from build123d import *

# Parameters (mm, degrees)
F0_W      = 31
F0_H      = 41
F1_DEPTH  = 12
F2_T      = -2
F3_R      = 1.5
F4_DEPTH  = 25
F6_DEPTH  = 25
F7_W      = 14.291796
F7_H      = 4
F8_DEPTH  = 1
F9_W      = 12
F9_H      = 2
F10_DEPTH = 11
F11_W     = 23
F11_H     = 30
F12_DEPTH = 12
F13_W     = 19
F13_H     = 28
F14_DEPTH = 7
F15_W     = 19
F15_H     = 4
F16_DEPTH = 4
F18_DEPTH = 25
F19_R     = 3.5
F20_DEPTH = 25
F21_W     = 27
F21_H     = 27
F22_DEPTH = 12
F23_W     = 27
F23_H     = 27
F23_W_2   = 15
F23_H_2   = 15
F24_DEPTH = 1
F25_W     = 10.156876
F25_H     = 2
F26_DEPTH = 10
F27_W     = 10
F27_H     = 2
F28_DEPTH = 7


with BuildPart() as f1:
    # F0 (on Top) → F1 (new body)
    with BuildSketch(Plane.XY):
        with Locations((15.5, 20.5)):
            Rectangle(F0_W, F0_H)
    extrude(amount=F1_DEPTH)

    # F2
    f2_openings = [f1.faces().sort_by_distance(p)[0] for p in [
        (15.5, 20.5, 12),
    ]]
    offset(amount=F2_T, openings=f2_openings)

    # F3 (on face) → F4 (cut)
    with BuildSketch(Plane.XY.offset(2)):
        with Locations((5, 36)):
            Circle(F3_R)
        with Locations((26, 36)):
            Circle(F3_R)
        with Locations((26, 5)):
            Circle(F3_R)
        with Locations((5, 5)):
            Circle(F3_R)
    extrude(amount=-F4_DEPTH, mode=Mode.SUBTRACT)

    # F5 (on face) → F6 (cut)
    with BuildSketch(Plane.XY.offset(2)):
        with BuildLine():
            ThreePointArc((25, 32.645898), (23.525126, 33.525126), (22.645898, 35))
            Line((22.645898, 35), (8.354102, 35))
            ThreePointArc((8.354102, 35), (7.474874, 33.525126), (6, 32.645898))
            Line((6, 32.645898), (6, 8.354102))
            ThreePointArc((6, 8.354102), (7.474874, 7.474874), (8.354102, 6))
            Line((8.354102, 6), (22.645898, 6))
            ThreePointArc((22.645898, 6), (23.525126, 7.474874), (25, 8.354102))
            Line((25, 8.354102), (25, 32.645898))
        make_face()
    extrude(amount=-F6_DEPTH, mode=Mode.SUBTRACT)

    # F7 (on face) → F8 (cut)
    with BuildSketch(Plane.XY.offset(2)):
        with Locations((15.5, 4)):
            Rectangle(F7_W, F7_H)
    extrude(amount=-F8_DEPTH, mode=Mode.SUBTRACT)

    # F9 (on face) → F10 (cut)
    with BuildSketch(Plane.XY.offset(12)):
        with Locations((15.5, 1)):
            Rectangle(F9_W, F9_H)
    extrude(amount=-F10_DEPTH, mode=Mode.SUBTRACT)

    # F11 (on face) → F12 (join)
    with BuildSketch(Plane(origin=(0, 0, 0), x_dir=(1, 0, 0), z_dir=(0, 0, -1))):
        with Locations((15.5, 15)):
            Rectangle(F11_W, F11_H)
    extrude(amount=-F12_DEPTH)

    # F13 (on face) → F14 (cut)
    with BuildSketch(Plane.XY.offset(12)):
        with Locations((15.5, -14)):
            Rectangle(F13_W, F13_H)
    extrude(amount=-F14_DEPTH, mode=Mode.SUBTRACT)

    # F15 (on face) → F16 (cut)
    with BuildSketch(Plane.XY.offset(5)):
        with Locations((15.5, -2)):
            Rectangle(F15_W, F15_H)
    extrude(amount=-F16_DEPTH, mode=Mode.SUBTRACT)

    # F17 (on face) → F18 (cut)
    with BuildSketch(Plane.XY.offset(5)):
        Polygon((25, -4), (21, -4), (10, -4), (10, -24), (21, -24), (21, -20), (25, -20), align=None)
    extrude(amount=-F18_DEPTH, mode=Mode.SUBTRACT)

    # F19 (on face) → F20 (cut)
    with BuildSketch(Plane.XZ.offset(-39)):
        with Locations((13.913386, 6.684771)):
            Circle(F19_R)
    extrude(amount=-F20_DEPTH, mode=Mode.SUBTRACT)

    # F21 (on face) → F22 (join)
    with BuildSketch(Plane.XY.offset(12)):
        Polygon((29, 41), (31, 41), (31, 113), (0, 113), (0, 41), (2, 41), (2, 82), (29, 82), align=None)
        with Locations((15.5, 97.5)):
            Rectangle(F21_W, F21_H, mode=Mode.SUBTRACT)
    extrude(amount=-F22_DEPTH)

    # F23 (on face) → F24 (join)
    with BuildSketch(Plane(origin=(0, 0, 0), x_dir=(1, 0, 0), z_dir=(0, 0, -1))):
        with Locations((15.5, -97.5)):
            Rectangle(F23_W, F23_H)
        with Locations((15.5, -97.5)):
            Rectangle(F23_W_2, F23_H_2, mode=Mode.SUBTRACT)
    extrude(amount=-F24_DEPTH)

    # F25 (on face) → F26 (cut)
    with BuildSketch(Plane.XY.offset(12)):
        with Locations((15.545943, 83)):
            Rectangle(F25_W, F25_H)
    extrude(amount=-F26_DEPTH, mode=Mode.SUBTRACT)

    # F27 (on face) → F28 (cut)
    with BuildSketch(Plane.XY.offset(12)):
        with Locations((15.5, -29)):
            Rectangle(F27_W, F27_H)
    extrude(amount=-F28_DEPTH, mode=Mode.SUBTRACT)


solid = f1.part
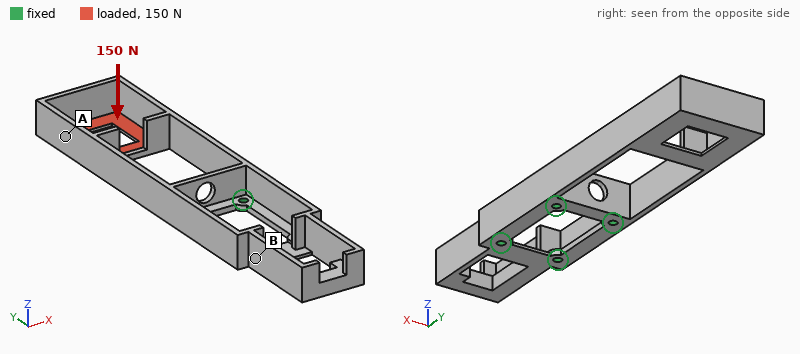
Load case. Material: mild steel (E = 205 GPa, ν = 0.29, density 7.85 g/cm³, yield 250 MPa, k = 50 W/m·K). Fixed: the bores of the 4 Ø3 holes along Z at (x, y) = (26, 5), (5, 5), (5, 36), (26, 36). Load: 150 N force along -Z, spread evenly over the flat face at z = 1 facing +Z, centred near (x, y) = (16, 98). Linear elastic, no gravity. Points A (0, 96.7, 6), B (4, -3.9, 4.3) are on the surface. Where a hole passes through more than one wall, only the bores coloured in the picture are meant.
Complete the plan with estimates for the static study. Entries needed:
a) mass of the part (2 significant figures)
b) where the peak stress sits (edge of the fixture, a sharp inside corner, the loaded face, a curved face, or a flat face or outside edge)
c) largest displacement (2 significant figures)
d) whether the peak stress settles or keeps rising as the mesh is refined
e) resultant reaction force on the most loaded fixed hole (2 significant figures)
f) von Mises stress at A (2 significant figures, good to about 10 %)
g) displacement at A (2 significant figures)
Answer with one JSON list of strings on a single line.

["90 g", "edge of the fixture", "0.17 mm", "keeps rising", "310 N", "14 MPa", "0.12 mm"]
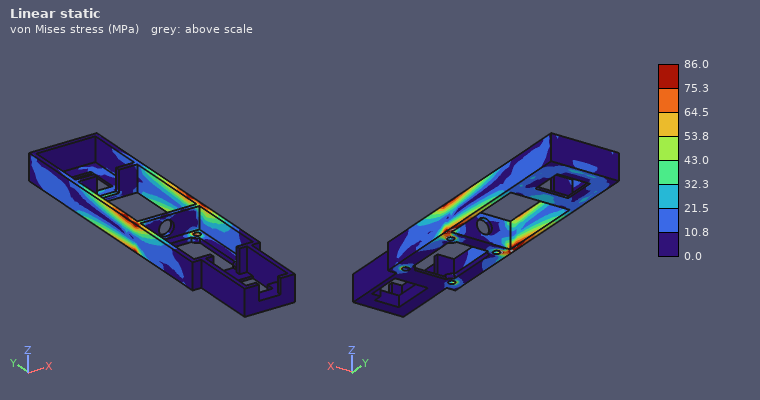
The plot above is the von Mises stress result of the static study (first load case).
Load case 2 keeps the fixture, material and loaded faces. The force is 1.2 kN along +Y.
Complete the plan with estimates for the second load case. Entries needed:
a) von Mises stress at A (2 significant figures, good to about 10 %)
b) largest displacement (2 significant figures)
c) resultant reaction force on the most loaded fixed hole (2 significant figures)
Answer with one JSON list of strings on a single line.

["15 MPa", "0.14 mm", "510 N"]
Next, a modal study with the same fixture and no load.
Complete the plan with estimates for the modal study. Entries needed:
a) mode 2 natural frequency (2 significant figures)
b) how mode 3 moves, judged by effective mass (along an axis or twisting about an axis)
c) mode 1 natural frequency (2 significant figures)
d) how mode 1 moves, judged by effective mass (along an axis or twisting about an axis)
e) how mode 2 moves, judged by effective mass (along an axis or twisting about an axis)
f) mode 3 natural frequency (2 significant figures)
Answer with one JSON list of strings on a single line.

["1000 Hz", "twisting about Y", "590 Hz", "along X", "along Z", "1600 Hz"]
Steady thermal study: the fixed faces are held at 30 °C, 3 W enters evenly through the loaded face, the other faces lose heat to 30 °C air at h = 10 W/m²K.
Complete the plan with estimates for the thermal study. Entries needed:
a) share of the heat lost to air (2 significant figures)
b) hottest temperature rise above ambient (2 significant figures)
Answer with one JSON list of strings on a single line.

["55 %", "41 K"]
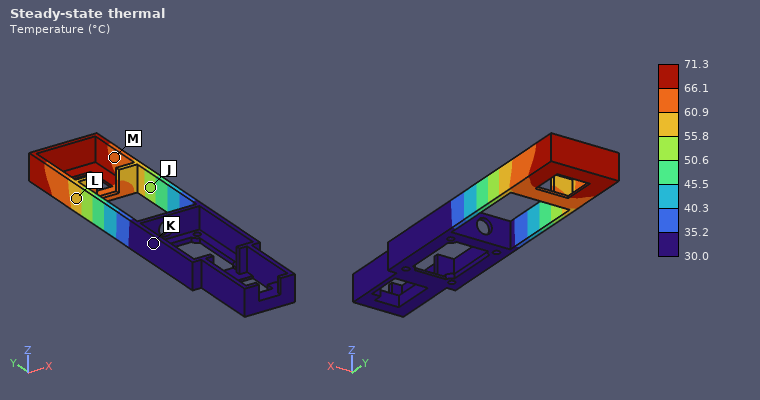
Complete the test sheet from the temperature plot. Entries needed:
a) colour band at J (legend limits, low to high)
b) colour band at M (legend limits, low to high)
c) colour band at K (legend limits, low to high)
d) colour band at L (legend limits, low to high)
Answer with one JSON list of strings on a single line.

["50.6 to 55.8 °C", "60.9 to 66.1 °C", "30.0 to 35.2 °C", "55.8 to 60.9 °C"]
